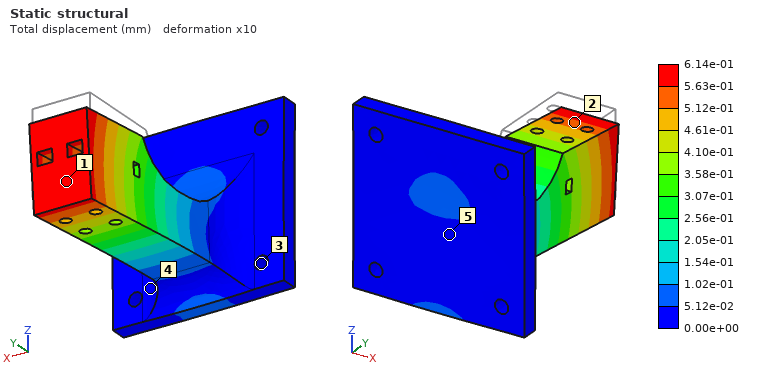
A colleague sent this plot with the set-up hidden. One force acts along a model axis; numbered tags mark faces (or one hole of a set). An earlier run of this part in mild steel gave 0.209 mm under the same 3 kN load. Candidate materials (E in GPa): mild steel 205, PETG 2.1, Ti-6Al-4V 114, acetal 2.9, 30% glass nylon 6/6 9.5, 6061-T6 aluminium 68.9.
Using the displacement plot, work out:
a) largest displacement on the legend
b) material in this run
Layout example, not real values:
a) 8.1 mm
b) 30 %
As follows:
a) 6.14e-01 mm
b) 6061-T6 aluminium
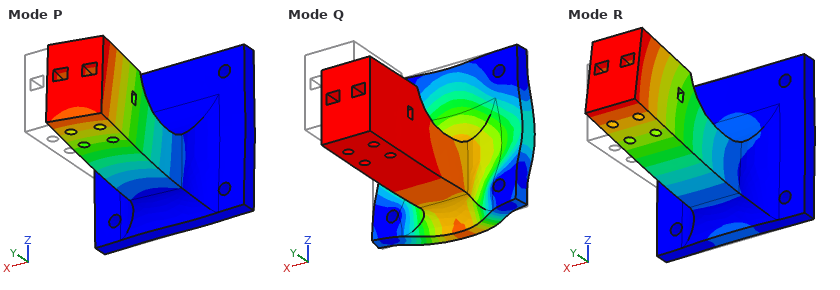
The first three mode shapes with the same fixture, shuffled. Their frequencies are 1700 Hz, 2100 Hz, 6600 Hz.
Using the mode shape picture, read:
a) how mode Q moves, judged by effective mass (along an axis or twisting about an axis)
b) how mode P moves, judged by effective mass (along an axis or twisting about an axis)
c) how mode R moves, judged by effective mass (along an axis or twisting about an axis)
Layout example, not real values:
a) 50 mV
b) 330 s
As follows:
a) along Y
b) along X
c) along Z
